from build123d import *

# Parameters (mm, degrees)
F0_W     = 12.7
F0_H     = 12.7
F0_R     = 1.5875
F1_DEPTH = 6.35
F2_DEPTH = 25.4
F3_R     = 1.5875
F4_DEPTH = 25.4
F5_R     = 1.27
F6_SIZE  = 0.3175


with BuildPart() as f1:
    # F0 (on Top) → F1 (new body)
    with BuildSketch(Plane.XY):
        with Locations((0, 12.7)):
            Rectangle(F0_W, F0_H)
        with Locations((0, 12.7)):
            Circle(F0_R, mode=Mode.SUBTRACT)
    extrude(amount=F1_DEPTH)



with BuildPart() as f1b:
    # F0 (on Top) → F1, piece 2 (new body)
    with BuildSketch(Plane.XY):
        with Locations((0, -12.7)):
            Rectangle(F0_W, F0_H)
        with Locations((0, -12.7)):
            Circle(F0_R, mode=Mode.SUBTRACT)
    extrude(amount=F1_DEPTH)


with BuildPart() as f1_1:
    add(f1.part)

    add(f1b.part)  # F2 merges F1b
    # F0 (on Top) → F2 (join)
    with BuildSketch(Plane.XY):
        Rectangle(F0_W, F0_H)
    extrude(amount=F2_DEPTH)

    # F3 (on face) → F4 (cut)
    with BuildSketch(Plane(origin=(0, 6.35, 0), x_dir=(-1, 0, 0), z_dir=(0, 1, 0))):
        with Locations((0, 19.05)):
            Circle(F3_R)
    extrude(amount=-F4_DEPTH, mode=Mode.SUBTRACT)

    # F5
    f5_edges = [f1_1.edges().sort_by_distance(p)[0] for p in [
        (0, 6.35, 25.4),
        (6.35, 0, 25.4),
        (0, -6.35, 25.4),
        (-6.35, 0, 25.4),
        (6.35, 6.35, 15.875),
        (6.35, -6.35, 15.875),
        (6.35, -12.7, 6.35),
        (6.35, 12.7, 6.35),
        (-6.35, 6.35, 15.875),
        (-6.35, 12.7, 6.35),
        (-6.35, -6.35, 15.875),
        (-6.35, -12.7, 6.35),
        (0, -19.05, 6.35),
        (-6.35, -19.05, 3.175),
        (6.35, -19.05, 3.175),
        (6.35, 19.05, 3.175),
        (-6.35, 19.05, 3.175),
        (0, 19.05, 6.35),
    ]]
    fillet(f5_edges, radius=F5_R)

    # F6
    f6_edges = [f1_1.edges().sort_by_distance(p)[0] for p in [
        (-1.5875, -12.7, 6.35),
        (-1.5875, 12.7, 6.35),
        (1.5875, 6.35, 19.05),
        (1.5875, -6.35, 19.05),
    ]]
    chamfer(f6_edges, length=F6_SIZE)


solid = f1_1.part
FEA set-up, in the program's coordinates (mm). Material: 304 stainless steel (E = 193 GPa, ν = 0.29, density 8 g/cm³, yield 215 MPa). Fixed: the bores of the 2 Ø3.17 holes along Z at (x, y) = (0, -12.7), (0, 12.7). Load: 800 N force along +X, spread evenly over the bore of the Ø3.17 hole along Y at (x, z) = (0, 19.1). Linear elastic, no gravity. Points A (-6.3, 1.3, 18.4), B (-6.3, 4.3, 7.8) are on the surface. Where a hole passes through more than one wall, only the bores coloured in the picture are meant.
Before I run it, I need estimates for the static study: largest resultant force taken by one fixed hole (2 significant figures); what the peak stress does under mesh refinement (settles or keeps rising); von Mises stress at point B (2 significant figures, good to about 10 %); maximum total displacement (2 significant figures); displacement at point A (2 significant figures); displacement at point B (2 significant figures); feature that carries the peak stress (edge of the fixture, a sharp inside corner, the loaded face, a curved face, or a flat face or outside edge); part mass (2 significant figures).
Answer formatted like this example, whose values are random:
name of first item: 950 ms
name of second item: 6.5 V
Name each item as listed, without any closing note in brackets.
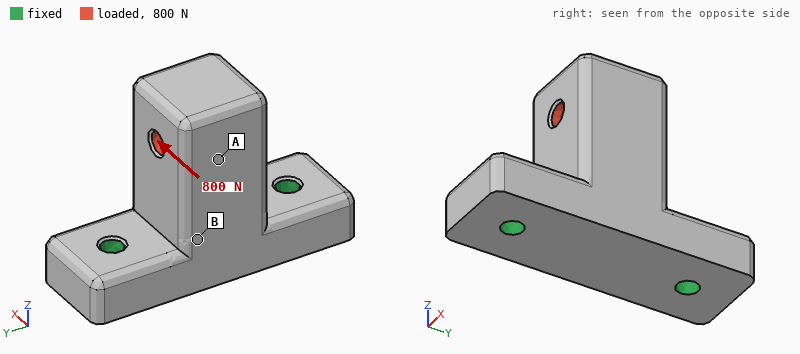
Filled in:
largest resultant force taken by one fixed hole: 400 N
what the peak stress does under mesh refinement: keeps rising
von Mises stress at point B: 29 MPa
maximum total displacement: 25 µm
displacement at point A: 18 µm
displacement at point B: 8.1 µm
feature that carries the peak stress: edge of the fixture
part mass: 47 g
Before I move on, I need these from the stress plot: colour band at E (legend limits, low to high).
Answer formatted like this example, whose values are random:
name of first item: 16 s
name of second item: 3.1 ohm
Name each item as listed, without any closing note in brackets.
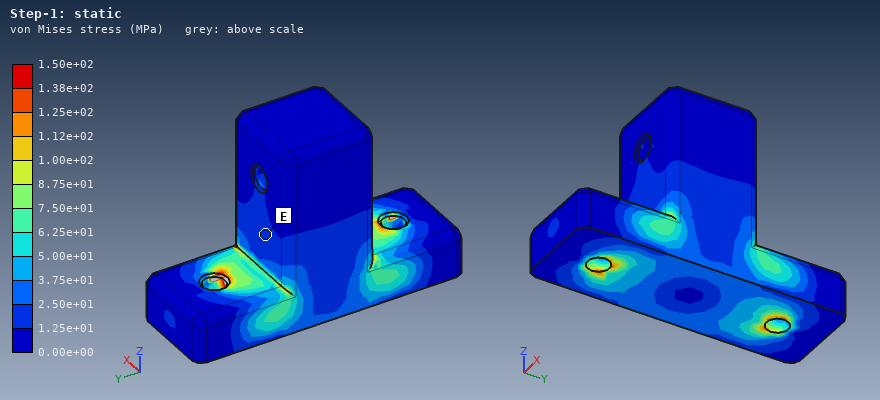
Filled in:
colour band at E: 1.25e+01 to 2.50e+01 MPa
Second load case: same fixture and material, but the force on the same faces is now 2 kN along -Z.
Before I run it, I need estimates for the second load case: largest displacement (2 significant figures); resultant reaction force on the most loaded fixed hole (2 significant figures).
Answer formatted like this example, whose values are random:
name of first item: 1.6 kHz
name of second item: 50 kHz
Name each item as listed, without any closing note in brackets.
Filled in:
largest displacement: 4.1 µm
resultant reaction force on the most loaded fixed hole: 1.0 kN
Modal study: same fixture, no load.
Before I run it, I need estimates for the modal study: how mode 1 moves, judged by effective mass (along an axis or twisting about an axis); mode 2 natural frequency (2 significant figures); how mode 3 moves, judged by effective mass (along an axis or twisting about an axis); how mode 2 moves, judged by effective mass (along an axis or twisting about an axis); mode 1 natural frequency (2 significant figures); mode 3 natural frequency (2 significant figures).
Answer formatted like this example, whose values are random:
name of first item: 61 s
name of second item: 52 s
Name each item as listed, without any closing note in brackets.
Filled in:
how mode 1 moves, judged by effective mass: along X
mode 2 natural frequency: 14 kHz
how mode 3 moves, judged by effective mass: along Z
how mode 2 moves, judged by effective mass: along Y
mode 1 natural frequency: 7800 Hz
mode 3 natural frequency: 22 kHz
